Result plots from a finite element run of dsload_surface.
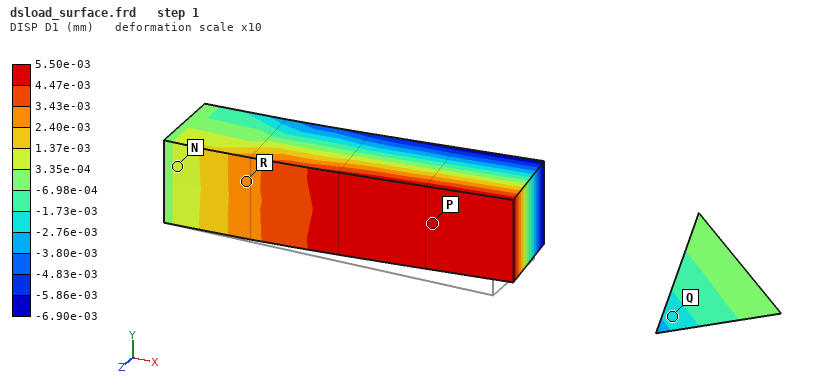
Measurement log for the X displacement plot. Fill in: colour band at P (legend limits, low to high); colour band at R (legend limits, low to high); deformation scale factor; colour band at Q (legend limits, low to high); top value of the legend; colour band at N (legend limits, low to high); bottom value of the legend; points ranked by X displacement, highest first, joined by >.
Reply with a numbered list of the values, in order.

1. 4.47e-03 to 5.50e-03 mm
2. 2.40e-03 to 3.43e-03 mm
3. 10
4. -2.76e-03 to -1.73e-03 mm
5. 5.50e-03 mm
6. 3.35e-04 to 1.37e-03 mm
7. -6.90e-03 mm
8. P > R > N > Q
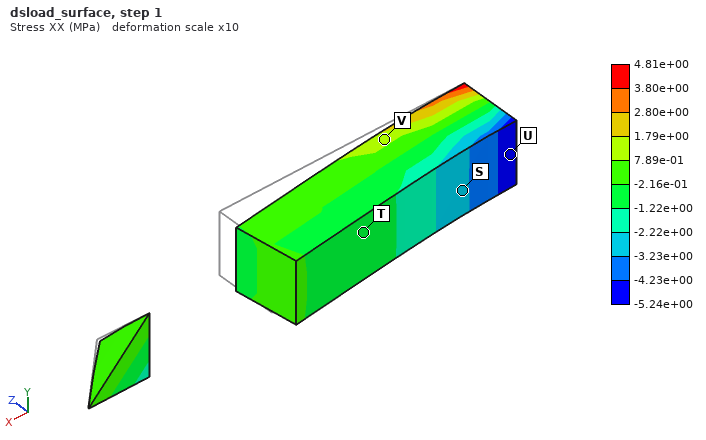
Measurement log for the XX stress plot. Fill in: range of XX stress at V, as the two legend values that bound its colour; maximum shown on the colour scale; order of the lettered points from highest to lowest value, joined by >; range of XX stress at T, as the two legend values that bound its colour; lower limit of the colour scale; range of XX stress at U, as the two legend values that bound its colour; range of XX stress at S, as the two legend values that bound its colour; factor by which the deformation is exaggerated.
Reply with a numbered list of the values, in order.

1. 7.89e-01 to 1.79e+00 MPa
2. 4.81e+00 MPa
3. V > T > S > U
4. -1.22e+00 to -2.16e-01 MPa
5. -5.24e+00 MPa
6. -5.24e+00 to -4.23e+00 MPa
7. -3.23e+00 to -2.22e+00 MPa
8. 10
